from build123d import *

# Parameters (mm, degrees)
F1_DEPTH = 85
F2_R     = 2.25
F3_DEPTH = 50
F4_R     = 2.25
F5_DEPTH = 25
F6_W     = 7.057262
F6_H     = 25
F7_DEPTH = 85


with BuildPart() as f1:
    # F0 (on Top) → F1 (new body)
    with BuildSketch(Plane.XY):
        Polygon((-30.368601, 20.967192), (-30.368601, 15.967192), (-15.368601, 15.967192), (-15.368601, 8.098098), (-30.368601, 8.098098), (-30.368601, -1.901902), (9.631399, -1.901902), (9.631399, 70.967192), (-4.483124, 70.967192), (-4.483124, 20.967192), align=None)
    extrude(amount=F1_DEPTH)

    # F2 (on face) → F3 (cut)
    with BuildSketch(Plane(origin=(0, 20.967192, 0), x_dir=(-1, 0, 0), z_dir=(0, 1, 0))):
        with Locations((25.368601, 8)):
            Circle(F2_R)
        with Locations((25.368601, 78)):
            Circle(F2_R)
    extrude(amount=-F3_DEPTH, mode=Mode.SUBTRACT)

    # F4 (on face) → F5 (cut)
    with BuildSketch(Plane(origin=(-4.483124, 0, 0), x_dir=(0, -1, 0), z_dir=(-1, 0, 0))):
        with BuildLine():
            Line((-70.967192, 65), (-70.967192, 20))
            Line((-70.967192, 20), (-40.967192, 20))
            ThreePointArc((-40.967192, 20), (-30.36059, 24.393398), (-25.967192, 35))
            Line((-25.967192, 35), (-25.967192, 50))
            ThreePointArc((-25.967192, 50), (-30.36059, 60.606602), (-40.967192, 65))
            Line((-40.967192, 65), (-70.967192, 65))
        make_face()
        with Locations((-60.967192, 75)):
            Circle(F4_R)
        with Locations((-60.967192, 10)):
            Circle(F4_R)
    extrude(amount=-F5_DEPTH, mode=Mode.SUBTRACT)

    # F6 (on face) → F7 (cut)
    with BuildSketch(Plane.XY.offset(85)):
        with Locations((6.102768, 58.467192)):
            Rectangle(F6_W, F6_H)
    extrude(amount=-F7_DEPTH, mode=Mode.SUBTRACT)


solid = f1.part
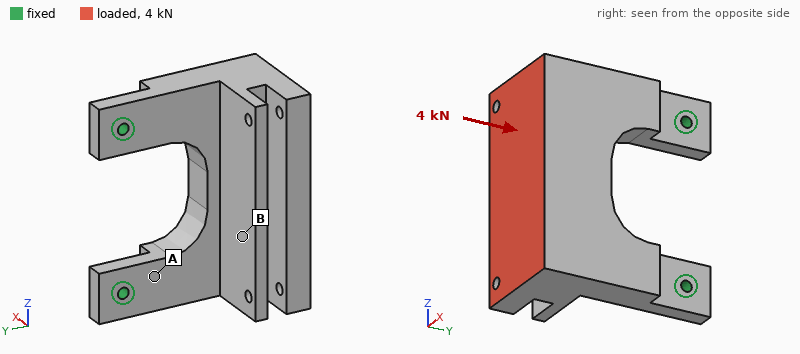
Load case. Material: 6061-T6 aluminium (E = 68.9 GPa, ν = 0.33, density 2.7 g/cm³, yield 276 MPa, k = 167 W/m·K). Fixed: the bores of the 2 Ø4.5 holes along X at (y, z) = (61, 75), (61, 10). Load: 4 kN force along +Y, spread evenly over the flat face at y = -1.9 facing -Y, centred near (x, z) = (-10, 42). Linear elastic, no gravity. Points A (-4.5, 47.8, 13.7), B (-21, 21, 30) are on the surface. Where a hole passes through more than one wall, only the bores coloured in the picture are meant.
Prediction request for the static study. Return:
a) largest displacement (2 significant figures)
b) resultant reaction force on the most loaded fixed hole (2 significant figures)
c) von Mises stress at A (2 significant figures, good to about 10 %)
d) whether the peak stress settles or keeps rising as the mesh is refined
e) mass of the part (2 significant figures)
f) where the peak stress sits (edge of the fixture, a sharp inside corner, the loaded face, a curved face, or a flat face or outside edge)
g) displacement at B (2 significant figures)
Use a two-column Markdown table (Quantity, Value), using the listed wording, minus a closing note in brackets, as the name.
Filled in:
| Quantity | Value |
|---|---|
| largest displacement | 0.60 mm |
| resultant reaction force on the most loaded fixed hole | 2.0 kN |
| von Mises stress at A | 120 MPa |
| whether the peak stress settles or keeps rising as the mesh is refined | keeps rising |
| mass of the part | 250 g |
| where the peak stress sits | edge of the fixture |
| displacement at B | 0.35 mm |
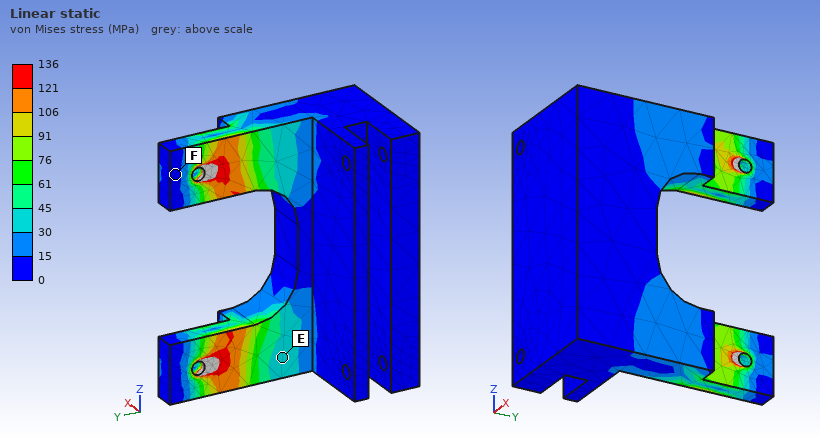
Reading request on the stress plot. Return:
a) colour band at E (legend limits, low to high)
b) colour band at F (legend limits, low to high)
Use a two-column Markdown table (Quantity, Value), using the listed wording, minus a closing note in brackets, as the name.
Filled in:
| Quantity | Value |
|---|---|
| colour band at E | 30 to 45 MPa |
| colour band at F | 0 to 15 MPa |
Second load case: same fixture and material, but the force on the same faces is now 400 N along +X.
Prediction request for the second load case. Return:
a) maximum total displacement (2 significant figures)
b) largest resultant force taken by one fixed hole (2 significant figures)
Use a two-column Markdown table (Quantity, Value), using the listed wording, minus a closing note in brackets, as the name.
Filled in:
| Quantity | Value |
|---|---|
| maximum total displacement | 0.32 mm |
| largest resultant force taken by one fixed hole | 200 N |
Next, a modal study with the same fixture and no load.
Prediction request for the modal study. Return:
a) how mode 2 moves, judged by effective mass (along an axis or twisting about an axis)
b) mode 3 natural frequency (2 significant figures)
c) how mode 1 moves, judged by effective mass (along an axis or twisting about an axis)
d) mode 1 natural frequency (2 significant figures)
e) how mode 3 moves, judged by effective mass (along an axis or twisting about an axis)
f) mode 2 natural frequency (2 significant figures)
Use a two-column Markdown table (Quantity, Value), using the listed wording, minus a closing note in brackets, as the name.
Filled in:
| Quantity | Value |
|---|---|
| how mode 2 moves, judged by effective mass | along Z |
| mode 3 natural frequency | 3000 Hz |
| how mode 1 moves, judged by effective mass | along X |
| mode 1 natural frequency | 510 Hz |
| how mode 3 moves, judged by effective mass | along Z |
| mode 2 natural frequency | 2000 Hz |
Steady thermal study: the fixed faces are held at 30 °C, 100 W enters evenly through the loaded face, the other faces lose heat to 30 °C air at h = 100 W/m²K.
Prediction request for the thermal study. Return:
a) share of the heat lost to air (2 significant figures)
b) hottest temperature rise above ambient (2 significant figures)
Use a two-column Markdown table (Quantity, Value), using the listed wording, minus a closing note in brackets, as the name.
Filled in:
| Quantity | Value |
|---|---|
| share of the heat lost to air | 51 % |
| hottest temperature rise above ambient | 40 K |
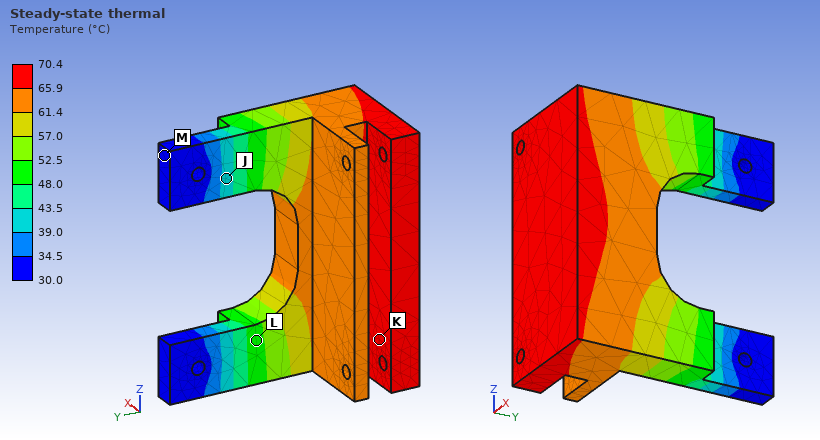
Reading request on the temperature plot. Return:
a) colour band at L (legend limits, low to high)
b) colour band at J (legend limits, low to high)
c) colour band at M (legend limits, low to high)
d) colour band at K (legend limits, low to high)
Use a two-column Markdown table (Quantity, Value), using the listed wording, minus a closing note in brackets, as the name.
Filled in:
| Quantity | Value |
|---|---|
| colour band at L | 48.0 to 52.5 °C |
| colour band at J | 39.0 to 43.5 °C |
| colour band at M | 30.0 to 34.5 °C |
| colour band at K | 65.9 to 70.4 °C |
